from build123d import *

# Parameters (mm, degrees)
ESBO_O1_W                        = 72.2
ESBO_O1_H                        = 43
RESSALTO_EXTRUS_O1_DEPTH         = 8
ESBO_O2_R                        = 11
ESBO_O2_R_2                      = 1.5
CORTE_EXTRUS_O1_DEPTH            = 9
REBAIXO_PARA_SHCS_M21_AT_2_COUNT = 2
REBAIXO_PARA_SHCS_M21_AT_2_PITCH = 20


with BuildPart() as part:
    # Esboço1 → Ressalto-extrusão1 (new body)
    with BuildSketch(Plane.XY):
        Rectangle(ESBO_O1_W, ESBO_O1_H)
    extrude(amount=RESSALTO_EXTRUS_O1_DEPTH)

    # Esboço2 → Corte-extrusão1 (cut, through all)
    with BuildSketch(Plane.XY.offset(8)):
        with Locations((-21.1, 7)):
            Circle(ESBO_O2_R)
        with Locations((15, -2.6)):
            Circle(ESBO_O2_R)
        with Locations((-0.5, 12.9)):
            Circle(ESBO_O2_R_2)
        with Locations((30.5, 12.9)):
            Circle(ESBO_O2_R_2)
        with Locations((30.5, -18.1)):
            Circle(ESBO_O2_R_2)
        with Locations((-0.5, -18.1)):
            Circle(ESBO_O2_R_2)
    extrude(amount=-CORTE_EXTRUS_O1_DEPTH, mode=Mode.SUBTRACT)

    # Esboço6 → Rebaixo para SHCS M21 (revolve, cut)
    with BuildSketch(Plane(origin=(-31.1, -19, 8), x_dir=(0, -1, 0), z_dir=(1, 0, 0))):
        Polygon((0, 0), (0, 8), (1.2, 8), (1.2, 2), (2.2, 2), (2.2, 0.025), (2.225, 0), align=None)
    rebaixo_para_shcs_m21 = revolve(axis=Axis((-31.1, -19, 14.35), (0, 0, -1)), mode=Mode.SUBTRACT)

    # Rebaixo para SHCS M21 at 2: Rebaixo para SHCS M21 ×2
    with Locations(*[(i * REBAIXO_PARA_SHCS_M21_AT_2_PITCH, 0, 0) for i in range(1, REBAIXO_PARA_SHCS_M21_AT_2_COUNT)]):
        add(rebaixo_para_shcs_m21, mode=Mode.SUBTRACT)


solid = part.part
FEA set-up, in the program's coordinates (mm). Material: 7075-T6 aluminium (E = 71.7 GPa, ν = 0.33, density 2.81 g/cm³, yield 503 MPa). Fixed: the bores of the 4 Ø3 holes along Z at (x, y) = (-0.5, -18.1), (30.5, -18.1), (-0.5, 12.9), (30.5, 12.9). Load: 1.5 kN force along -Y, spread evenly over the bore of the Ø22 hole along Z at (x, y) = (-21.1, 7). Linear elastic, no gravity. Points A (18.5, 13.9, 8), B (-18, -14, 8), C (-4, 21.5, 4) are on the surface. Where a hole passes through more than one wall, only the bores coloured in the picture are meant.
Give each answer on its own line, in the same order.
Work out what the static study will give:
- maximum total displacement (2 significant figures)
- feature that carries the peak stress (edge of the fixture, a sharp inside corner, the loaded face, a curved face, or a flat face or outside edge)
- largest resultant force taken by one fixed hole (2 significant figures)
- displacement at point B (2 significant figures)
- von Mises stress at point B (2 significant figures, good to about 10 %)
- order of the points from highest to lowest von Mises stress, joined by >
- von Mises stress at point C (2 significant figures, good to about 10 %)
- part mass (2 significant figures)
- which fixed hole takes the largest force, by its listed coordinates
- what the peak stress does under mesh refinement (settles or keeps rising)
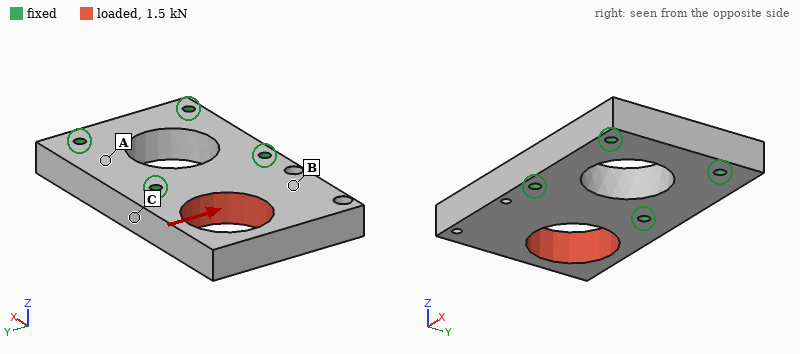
24 µm
a sharp inside corner
1.2 kN
7.4 µm
9.4 MPa
C > B > A
18 MPa
52 g
(-0.5, 12.9)
keeps rising
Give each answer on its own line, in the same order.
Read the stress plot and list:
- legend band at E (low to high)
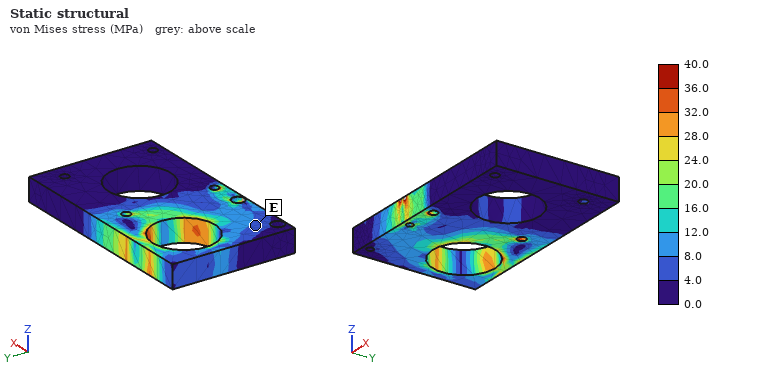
4.0 to 8.0 MPa
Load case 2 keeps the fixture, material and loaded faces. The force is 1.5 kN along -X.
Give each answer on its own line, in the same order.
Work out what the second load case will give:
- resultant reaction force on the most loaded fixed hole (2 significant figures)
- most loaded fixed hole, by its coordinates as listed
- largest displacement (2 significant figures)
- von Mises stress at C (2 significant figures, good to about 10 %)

1.0 kN
(-0.5, 12.9)
13 µm
13 MPa
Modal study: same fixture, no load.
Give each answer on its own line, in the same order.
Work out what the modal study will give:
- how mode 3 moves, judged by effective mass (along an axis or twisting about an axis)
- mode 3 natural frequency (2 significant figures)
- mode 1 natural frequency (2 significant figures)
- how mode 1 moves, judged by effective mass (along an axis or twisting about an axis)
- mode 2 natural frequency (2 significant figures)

along Y
11 kHz
4200 Hz
along Z
8100 Hz
